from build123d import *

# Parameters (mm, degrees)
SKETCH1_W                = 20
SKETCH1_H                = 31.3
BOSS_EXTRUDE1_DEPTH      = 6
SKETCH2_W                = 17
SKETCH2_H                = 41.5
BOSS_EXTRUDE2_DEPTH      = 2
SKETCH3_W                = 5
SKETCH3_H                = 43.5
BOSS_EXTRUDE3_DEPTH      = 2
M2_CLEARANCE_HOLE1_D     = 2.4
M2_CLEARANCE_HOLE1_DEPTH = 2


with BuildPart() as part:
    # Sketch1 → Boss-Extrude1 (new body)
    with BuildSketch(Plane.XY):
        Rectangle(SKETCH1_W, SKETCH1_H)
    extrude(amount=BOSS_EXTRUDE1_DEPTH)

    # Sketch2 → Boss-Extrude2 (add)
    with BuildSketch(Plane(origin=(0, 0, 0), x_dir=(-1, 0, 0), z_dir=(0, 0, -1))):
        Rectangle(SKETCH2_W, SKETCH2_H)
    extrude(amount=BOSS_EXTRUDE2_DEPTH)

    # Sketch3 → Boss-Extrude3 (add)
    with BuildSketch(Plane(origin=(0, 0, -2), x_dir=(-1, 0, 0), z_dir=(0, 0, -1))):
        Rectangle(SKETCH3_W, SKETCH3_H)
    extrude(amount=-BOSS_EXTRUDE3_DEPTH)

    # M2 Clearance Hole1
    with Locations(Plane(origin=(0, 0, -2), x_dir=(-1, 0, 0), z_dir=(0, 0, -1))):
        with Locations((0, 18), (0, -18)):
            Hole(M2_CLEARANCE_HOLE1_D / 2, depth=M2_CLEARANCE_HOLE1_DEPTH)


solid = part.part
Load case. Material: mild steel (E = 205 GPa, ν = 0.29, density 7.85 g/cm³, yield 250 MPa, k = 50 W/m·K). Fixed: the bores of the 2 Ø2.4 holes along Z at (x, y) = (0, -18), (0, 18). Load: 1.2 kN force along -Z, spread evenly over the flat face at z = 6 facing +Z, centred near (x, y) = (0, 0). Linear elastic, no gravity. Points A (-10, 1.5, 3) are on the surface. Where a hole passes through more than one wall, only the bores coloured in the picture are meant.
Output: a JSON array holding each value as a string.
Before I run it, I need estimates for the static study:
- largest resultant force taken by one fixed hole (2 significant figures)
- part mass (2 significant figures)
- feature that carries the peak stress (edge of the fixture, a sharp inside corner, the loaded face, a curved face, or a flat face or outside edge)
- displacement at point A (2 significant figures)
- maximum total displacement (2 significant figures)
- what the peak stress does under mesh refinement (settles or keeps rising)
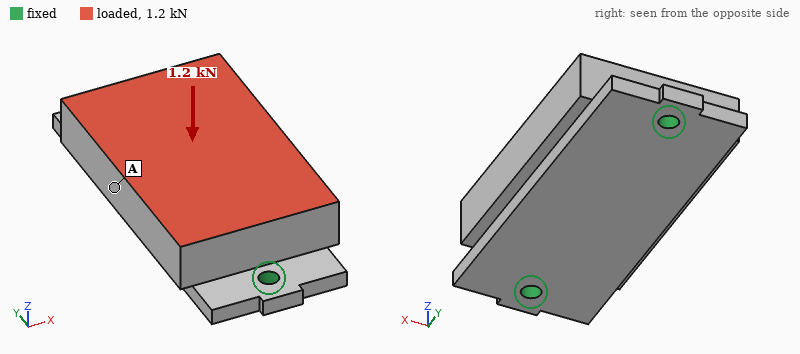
["770 N", "41 g", "edge of the fixture", "5.7 µm", "5.7 µm", "keeps rising"]
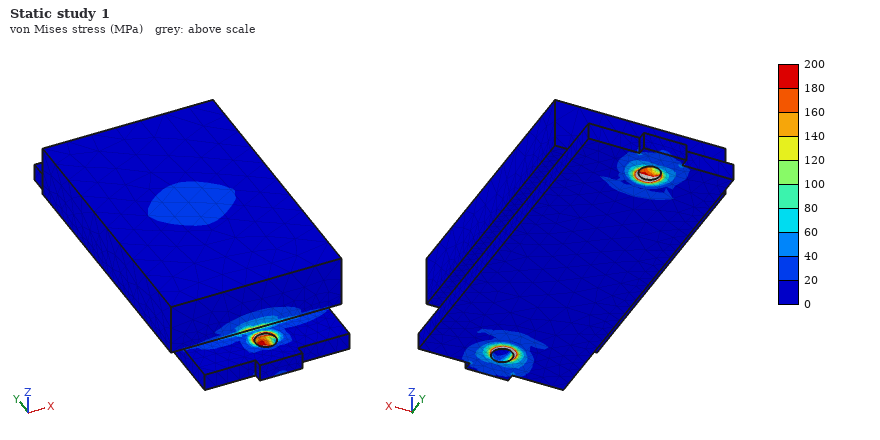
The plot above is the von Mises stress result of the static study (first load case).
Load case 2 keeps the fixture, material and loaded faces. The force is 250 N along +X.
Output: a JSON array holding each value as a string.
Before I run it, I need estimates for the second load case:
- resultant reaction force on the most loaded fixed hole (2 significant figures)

["130 N"]
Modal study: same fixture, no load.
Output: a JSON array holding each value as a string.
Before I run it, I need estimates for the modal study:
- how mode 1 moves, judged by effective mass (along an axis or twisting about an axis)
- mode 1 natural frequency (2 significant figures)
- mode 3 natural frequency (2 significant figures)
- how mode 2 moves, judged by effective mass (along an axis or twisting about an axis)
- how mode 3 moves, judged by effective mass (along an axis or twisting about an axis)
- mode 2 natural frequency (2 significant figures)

["along X", "5400 Hz", "22 kHz", "along Z", "along X", "13 kHz"]
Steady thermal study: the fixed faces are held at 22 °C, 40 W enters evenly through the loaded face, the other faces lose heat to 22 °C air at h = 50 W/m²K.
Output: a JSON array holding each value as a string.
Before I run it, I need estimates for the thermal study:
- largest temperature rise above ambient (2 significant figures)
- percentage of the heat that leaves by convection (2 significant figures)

["83 K", "14 %"]
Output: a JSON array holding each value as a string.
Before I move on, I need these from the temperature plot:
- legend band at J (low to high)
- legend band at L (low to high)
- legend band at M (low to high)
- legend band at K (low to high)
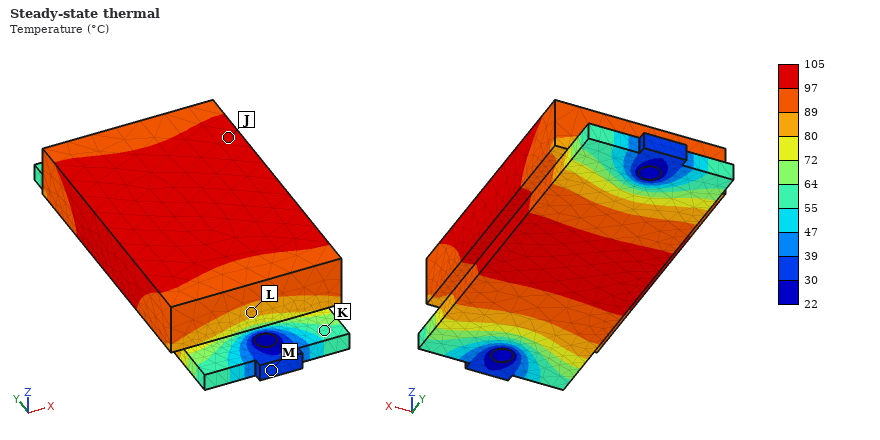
["97 to 105 °C", "80 to 89 °C", "30 to 39 °C", "55 to 64 °C"]
